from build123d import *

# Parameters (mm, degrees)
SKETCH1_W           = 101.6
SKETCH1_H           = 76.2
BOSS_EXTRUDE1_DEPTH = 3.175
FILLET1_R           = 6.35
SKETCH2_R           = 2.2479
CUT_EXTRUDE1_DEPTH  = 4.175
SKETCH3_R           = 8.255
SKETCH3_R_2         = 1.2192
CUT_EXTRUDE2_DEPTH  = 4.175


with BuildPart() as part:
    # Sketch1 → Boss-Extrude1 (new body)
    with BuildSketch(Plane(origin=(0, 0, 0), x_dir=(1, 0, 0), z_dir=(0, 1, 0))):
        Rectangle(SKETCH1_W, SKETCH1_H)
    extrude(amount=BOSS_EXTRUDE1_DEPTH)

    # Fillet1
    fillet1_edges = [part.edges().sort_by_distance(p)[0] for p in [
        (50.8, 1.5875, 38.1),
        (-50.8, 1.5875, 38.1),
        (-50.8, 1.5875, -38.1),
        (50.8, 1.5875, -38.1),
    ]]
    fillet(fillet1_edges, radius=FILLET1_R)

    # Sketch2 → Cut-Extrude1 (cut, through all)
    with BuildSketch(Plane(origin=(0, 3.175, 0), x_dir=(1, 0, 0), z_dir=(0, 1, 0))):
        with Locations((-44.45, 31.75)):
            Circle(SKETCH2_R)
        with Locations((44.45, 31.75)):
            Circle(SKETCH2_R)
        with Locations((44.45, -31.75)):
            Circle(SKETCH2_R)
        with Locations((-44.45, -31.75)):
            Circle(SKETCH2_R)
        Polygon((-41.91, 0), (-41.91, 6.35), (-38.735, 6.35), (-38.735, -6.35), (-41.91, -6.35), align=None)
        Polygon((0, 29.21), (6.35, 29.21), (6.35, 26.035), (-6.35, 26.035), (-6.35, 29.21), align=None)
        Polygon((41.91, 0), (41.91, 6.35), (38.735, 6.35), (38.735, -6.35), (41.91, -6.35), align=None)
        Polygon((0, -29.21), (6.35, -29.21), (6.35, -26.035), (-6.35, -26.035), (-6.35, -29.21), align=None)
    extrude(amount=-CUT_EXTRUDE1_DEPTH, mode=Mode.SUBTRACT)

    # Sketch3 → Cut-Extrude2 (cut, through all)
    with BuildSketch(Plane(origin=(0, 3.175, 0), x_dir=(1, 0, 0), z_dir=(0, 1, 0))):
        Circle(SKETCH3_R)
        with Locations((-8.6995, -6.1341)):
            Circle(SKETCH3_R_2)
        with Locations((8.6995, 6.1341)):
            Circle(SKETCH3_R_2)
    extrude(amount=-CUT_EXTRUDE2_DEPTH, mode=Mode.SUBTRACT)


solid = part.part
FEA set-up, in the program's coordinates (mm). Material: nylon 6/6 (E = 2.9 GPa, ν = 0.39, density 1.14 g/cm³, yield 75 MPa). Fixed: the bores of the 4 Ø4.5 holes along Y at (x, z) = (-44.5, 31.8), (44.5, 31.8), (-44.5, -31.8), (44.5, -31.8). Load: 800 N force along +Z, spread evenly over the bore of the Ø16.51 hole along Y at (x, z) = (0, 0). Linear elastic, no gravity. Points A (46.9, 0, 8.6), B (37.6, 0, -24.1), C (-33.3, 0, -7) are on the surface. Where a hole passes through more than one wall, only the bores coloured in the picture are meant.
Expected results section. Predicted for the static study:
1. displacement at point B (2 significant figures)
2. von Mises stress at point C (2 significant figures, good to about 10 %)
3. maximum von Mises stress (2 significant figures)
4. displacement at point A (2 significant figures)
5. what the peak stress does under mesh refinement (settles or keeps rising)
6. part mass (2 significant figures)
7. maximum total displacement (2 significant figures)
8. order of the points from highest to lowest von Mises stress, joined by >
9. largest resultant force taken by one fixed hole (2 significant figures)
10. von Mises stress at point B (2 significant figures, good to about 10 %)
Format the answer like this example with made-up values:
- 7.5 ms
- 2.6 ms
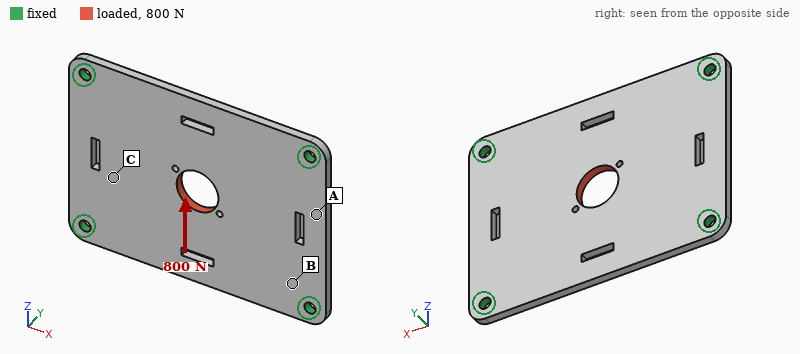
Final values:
- 0.022 mm
- 2.7 MPa
- 17 MPa
- 0.016 mm
- settles
- 26 g
- 0.11 mm
- B > C > A
- 250 N
- 4.8 MPa
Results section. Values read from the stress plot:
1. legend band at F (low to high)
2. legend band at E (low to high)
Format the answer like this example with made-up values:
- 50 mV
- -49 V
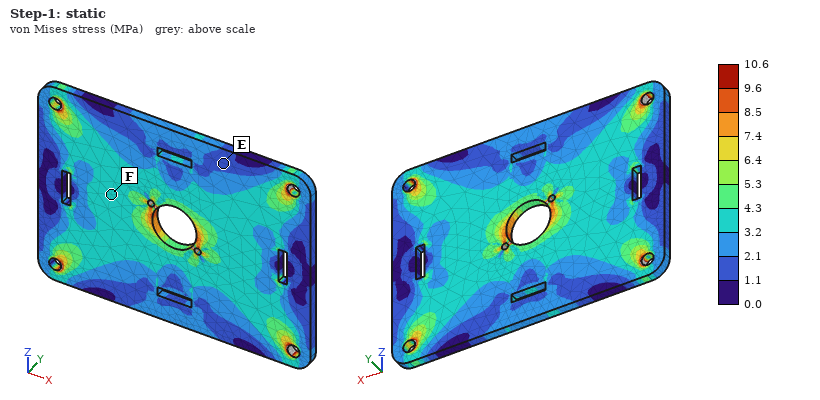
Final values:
- 3.2 to 4.3 MPa
- 1.1 to 2.1 MPa
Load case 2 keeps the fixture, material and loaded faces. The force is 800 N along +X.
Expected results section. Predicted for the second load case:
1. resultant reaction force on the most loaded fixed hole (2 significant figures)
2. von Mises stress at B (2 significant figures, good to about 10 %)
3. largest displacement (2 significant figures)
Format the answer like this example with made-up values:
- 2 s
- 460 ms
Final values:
- 220 N
- 3.9 MPa
- 74 µm
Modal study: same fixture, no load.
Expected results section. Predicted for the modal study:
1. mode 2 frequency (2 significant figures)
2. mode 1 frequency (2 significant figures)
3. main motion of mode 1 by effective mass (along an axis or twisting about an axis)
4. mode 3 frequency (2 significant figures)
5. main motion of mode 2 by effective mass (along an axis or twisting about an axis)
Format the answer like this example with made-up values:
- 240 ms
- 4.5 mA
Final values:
- 840 Hz
- 540 Hz
- along Y
- 1200 Hz
- twisting about X
